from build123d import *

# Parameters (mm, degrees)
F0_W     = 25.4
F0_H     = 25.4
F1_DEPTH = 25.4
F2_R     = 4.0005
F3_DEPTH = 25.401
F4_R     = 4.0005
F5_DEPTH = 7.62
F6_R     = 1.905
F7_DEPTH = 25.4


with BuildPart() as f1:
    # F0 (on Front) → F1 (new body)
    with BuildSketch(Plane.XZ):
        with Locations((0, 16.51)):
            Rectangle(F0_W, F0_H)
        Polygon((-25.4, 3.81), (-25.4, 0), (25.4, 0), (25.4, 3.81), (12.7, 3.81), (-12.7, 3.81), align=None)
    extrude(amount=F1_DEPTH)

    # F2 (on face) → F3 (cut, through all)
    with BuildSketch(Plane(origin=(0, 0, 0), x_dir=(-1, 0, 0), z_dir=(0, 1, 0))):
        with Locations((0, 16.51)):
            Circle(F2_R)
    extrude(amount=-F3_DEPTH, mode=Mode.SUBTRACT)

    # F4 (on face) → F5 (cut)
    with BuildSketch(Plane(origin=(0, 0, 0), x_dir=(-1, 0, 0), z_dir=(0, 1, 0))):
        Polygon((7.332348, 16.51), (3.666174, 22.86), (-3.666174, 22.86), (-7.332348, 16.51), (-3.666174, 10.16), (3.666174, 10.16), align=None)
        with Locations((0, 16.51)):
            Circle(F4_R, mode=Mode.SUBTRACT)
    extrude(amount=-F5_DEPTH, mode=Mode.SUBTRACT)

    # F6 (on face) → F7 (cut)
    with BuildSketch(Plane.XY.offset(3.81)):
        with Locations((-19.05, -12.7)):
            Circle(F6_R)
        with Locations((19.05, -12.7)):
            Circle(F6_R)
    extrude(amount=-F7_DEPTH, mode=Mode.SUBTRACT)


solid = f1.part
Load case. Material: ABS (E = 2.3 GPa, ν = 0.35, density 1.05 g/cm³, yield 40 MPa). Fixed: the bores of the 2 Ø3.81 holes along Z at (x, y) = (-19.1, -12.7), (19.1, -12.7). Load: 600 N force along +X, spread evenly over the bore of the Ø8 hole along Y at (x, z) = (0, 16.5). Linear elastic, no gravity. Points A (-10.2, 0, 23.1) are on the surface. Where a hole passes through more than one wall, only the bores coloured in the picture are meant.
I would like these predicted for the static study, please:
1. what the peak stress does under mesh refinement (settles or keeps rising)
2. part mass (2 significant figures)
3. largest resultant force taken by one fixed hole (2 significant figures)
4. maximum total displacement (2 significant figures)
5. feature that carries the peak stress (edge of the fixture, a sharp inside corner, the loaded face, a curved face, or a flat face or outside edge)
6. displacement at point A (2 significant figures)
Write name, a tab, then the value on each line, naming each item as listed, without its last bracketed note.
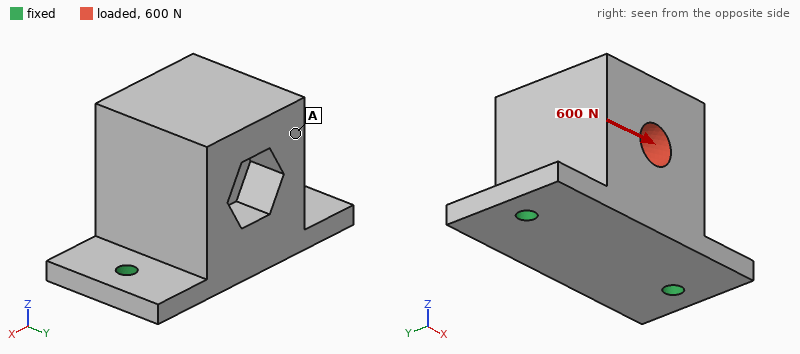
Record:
what the peak stress does under mesh refinement	keeps rising
part mass	20 g
largest resultant force taken by one fixed hole	410 N
maximum total displacement	0.27 mm
feature that carries the peak stress	edge of the fixture
displacement at point A	0.20 mm
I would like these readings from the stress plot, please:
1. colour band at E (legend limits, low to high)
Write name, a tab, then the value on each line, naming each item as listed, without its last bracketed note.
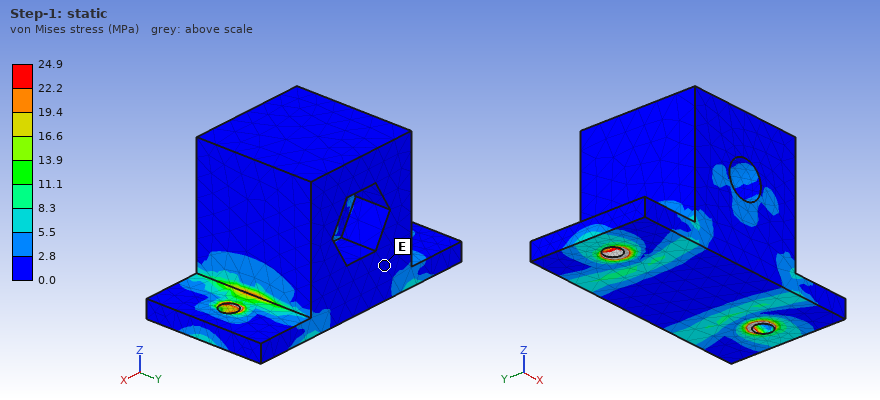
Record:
colour band at E	0.0 to 2.8 MPa
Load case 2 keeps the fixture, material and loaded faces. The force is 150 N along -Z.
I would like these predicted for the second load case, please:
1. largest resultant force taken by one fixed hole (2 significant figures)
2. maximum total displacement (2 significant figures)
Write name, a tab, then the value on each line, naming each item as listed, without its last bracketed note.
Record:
largest resultant force taken by one fixed hole	82 N
maximum total displacement	0.17 mm
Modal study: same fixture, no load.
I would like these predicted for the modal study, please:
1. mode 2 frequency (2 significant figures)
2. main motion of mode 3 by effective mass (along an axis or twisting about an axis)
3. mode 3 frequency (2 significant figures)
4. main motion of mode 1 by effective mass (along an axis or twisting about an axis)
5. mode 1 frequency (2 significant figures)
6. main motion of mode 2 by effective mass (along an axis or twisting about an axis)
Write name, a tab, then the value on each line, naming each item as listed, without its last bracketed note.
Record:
mode 2 frequency	2200 Hz
main motion of mode 3 by effective mass	along Z
mode 3 frequency	2500 Hz
main motion of mode 1 by effective mass	along Y
mode 1 frequency	740 Hz
main motion of mode 2 by effective mass	along X
